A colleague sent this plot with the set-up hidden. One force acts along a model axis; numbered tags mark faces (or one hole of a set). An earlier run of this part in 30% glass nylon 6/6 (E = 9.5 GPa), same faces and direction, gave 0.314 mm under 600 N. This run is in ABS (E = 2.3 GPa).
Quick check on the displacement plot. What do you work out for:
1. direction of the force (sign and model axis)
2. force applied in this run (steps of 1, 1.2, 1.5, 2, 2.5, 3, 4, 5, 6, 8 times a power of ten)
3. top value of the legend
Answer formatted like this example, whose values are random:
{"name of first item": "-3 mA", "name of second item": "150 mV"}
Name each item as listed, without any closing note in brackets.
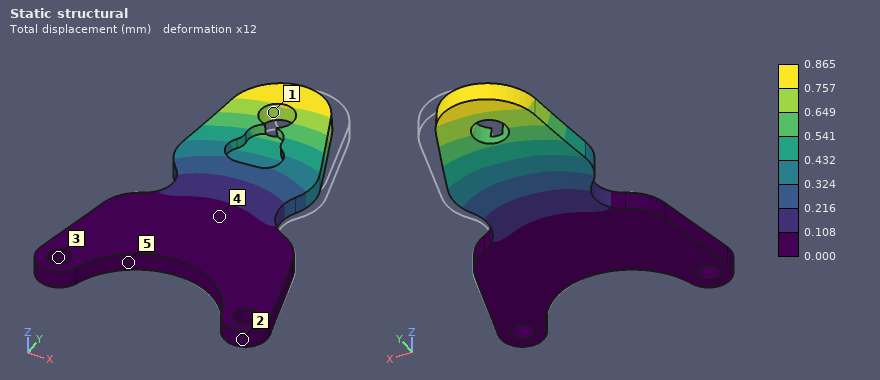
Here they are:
{"direction of the force": "-X", "force applied in this run": "400 N", "top value of the legend": "0.865 mm"}
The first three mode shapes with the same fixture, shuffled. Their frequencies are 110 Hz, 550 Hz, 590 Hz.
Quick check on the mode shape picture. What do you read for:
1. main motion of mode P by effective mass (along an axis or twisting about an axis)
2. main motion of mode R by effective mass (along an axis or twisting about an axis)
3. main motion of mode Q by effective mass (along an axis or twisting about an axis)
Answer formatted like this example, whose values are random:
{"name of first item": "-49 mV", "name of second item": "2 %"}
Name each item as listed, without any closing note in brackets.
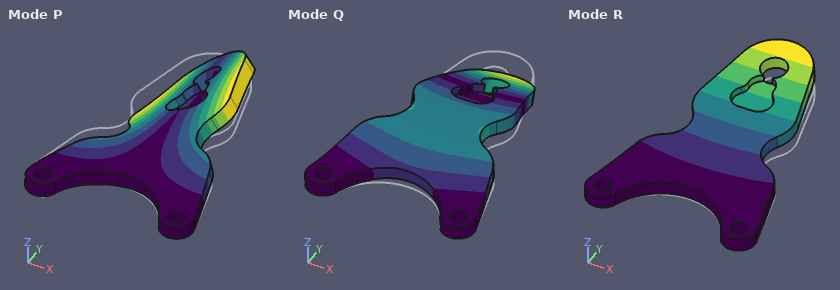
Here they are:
{"main motion of mode P by effective mass": "twisting about Y", "main motion of mode R by effective mass": "along Z", "main motion of mode Q by effective mass": "along Z"}
